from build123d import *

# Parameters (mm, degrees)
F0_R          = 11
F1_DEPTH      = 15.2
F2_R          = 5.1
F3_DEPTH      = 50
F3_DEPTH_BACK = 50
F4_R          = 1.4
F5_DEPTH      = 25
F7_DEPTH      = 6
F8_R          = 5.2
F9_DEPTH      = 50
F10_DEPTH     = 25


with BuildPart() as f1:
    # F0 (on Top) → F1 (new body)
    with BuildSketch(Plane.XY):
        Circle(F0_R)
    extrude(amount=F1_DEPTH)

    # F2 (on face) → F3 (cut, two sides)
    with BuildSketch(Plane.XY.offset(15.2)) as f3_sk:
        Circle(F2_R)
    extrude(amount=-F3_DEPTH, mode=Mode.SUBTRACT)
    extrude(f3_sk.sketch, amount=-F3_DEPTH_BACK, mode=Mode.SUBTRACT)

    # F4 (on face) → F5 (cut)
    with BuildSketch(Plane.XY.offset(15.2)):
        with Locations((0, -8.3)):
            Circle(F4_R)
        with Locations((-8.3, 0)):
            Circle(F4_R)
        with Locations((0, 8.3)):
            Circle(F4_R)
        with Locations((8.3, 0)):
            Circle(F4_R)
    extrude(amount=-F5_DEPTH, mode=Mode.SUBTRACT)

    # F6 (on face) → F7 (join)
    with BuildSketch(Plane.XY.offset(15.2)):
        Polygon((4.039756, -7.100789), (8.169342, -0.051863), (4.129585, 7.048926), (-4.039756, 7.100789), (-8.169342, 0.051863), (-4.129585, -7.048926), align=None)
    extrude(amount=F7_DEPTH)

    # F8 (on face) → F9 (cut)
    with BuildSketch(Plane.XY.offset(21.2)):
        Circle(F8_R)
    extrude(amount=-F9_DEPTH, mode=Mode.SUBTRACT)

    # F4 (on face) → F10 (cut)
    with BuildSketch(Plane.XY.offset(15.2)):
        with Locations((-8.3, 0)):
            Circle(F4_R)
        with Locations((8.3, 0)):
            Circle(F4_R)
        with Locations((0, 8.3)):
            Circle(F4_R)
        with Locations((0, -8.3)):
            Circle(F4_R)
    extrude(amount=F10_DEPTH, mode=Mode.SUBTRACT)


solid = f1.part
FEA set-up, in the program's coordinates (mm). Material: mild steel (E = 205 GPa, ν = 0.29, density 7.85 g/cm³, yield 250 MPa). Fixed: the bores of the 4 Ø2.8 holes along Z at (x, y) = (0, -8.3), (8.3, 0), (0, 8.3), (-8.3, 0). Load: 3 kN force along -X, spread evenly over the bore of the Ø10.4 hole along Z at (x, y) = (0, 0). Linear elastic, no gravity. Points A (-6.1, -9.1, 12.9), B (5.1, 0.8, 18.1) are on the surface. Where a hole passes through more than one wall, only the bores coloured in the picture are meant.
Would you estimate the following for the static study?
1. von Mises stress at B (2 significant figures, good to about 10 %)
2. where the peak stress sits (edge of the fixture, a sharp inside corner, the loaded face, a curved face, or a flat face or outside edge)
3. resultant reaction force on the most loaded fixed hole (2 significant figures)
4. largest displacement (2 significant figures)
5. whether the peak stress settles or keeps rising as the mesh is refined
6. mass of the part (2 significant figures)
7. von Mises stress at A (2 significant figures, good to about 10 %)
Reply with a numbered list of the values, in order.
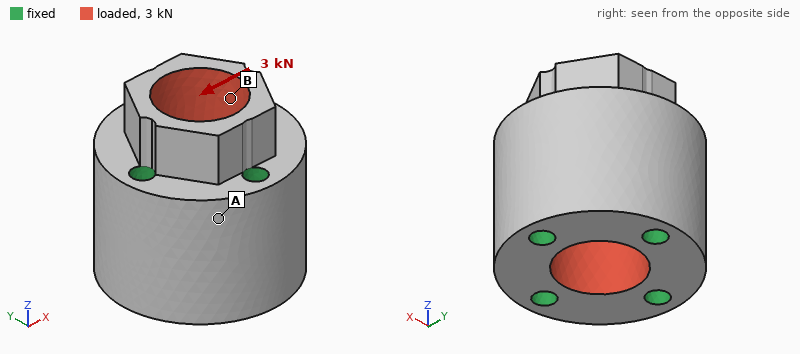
1. 13 MPa
2. edge of the fixture
3. 770 N
4. 1.6 µm
5. keeps rising
6. 36 g
7. 4.6 MPa
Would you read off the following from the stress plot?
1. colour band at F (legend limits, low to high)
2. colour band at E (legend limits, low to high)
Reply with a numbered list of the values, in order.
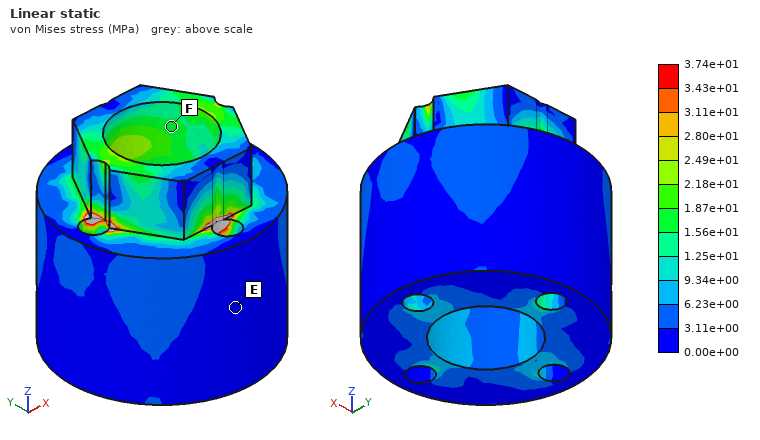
1. 1.56e+01 to 1.87e+01 MPa
2. 0.00e+00 to 3.11e+00 MPa
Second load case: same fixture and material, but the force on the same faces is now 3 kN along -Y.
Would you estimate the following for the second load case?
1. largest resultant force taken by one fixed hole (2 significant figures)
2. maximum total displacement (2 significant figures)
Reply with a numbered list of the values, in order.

1. 770 N
2. 1.6 µm
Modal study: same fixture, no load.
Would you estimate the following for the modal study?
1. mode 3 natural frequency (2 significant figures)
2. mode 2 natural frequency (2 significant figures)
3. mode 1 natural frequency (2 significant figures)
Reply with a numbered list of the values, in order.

1. 76 kHz
2. 75 kHz
3. 67 kHz
